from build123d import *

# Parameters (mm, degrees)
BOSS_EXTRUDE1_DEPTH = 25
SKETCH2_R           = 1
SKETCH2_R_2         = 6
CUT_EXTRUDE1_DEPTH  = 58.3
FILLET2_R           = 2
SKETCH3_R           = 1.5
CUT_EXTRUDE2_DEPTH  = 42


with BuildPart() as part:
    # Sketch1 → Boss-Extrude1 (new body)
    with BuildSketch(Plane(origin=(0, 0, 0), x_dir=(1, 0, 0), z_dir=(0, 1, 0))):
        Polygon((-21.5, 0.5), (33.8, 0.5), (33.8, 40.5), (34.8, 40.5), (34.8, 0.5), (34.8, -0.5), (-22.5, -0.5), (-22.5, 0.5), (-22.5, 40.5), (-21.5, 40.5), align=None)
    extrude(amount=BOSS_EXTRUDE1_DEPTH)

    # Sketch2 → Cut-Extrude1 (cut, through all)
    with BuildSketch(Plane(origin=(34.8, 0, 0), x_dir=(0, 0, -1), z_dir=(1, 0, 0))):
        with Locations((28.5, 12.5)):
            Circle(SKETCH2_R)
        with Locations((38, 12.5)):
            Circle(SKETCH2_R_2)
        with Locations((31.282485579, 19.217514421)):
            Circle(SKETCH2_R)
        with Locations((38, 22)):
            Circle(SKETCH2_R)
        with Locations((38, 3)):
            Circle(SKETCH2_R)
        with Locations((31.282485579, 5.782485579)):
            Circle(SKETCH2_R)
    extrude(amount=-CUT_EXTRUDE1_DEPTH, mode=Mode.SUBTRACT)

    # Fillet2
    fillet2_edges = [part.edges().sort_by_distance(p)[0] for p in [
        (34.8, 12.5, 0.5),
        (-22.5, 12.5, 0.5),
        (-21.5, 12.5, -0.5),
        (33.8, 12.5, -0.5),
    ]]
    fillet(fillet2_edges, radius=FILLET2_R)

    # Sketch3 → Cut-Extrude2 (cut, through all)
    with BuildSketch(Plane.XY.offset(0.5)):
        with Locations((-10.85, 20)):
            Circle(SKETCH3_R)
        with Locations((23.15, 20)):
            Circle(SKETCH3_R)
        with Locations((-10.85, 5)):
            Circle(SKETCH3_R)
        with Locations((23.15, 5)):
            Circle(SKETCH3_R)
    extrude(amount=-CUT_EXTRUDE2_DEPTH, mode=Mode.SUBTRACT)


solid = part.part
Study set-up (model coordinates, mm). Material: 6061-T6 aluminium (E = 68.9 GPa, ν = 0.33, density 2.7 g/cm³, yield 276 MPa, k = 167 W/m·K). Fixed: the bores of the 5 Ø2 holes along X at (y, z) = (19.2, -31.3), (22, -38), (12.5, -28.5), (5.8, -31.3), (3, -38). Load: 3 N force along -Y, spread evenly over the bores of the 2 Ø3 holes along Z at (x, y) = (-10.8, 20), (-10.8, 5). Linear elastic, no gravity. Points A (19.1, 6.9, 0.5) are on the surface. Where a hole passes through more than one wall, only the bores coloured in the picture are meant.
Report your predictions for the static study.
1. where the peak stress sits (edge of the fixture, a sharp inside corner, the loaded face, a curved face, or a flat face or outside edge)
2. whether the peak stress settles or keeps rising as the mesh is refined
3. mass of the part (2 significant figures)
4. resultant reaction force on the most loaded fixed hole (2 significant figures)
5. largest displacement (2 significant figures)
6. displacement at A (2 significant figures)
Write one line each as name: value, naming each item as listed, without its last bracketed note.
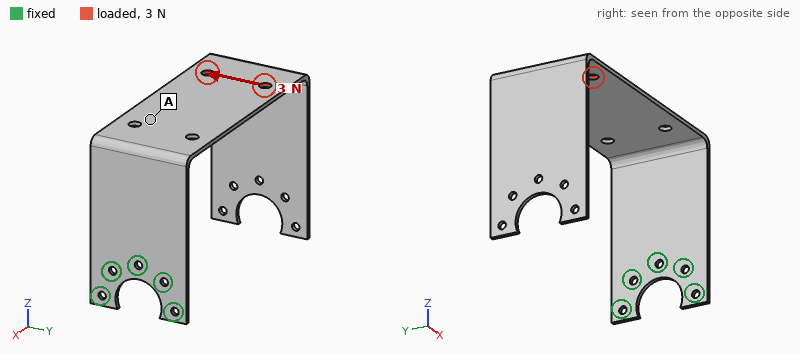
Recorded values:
where the peak stress sits: edge of the fixture
whether the peak stress settles or keeps rising as the mesh is refined: keeps rising
mass of the part: 8.6 g
resultant reaction force on the most loaded fixed hole: 8.9 N
largest displacement: 0.87 mm
displacement at A: 0.22 mm
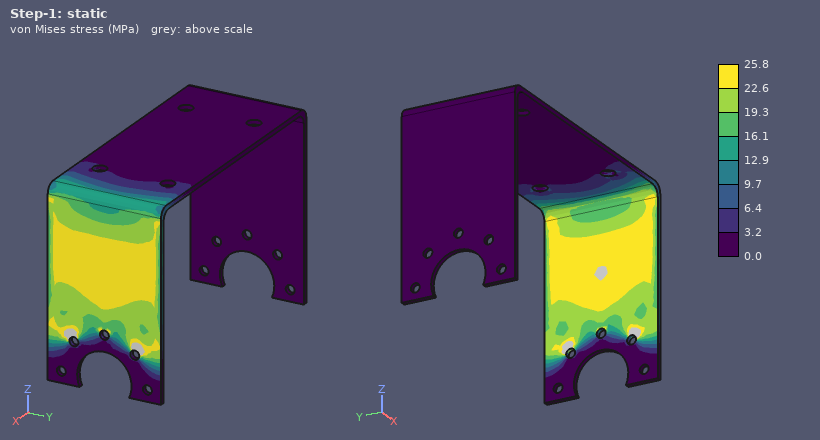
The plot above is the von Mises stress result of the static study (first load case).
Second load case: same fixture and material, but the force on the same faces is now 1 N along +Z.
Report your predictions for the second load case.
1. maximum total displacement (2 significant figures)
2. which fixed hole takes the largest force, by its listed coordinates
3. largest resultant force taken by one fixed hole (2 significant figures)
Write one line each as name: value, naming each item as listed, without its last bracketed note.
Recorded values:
maximum total displacement: 0.88 mm
which fixed hole takes the largest force, by its listed coordinates: (12.5, -28.5)
largest resultant force taken by one fixed hole: 3.8 N
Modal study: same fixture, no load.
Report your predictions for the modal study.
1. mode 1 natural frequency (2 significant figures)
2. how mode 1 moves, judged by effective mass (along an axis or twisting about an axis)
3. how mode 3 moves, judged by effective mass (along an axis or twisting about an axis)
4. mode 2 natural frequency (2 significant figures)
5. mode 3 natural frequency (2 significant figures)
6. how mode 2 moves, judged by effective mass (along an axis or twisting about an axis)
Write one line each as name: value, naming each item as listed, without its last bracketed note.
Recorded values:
mode 1 natural frequency: 82 Hz
how mode 1 moves, judged by effective mass: along Z
how mode 3 moves, judged by effective mass: along X
mode 2 natural frequency: 130 Hz
mode 3 natural frequency: 260 Hz
how mode 2 moves, judged by effective mass: along Y
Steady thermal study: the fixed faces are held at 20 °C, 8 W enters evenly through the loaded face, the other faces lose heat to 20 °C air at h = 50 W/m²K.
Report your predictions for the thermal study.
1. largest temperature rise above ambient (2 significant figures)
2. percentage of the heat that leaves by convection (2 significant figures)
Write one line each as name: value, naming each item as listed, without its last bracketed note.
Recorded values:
largest temperature rise above ambient: 43 K
percentage of the heat that leaves by convection: 83 %
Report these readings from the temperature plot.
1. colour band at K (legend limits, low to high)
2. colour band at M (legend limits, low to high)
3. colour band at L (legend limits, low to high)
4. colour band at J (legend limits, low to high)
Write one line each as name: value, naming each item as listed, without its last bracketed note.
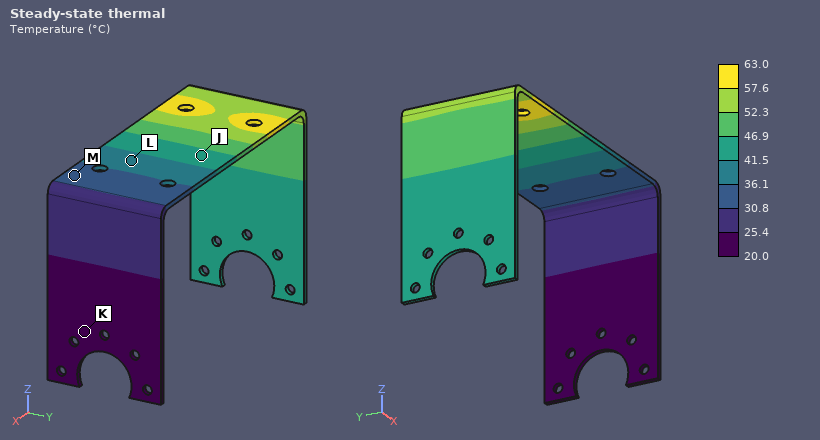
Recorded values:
colour band at K: 20.0 to 25.4 °C
colour band at M: 30.8 to 36.1 °C
colour band at L: 36.1 to 41.5 °C
colour band at J: 41.5 to 46.9 °C
